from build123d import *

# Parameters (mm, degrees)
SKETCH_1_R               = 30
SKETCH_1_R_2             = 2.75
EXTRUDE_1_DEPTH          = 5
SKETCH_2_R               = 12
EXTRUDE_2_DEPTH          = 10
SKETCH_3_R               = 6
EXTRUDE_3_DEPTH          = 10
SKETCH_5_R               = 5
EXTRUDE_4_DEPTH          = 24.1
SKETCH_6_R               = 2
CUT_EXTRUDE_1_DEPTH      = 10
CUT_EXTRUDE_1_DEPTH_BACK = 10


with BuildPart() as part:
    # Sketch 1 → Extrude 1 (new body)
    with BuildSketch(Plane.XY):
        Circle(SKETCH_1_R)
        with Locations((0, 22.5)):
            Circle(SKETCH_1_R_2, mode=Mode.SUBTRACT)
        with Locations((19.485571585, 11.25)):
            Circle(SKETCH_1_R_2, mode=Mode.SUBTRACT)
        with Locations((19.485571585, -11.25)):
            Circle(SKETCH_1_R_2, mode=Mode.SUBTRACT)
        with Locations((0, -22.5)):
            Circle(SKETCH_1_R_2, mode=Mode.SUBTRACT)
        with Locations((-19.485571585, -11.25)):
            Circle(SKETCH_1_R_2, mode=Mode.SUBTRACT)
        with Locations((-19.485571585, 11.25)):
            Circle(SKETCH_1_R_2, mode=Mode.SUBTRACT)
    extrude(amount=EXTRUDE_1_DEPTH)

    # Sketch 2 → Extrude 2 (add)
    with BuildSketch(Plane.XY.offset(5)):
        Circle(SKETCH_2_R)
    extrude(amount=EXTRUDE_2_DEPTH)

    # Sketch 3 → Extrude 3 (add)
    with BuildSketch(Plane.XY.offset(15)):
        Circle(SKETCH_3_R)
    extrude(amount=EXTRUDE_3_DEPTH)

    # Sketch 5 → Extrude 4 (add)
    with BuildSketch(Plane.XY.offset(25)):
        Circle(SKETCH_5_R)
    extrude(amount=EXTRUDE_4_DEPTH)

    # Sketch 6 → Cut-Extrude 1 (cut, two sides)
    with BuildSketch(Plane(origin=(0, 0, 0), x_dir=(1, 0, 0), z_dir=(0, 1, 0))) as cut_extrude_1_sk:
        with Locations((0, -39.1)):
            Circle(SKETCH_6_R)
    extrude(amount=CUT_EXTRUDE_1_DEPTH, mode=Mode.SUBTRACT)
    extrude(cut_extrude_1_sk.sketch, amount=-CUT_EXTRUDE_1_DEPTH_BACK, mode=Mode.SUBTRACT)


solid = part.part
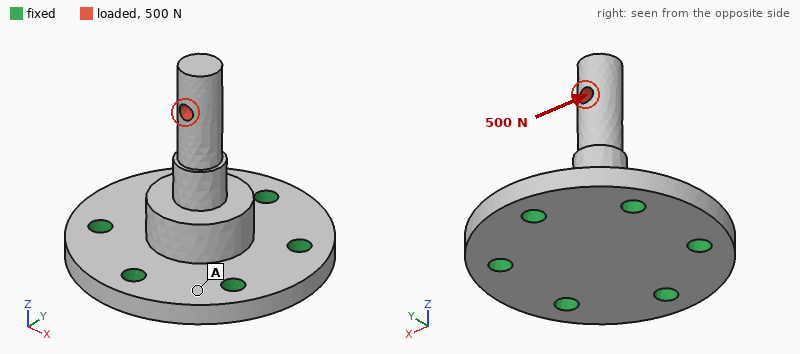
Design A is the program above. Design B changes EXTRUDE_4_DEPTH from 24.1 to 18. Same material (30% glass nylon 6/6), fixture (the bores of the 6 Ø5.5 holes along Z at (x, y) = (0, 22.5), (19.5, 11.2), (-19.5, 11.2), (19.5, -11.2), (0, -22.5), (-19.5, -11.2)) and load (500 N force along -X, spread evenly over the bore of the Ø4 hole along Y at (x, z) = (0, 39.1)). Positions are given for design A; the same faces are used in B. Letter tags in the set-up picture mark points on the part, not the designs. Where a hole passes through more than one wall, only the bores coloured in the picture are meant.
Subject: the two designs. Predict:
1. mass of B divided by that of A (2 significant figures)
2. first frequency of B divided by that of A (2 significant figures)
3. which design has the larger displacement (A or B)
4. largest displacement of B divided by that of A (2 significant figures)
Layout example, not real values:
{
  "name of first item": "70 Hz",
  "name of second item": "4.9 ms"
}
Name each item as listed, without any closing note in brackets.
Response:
{
  "mass of B divided by that of A": "0.98",
  "first frequency of B divided by that of A": "1.4",
  "which design has the larger displacement": "A",
  "largest displacement of B divided by that of A": "0.81"
}
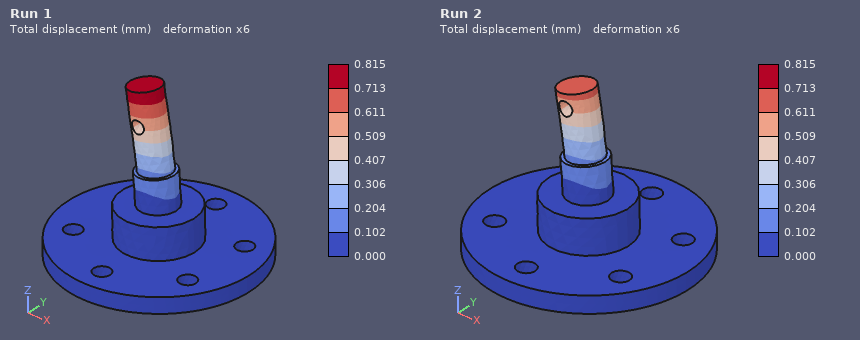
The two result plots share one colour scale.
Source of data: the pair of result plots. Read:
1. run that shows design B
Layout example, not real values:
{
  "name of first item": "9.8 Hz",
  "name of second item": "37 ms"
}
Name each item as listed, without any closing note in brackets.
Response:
{
  "run that shows design B": "Run 2"
}
